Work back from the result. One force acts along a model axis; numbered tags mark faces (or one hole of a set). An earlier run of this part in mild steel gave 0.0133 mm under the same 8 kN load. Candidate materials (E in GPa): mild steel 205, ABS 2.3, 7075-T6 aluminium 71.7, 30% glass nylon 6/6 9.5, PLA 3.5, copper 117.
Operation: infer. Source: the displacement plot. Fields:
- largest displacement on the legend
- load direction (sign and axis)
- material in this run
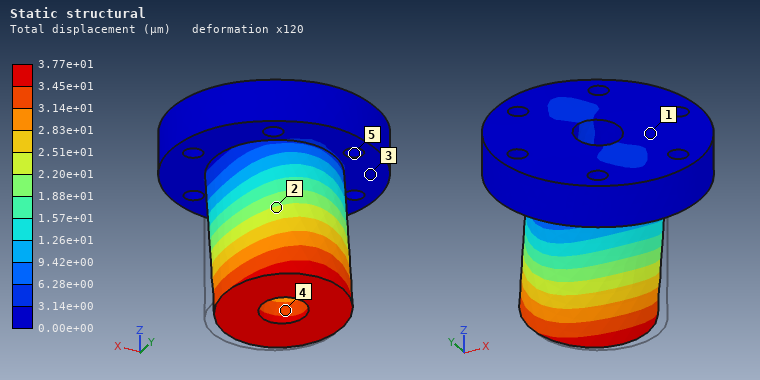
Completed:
3.77e+01 µm
+Y
7075-T6 aluminium
